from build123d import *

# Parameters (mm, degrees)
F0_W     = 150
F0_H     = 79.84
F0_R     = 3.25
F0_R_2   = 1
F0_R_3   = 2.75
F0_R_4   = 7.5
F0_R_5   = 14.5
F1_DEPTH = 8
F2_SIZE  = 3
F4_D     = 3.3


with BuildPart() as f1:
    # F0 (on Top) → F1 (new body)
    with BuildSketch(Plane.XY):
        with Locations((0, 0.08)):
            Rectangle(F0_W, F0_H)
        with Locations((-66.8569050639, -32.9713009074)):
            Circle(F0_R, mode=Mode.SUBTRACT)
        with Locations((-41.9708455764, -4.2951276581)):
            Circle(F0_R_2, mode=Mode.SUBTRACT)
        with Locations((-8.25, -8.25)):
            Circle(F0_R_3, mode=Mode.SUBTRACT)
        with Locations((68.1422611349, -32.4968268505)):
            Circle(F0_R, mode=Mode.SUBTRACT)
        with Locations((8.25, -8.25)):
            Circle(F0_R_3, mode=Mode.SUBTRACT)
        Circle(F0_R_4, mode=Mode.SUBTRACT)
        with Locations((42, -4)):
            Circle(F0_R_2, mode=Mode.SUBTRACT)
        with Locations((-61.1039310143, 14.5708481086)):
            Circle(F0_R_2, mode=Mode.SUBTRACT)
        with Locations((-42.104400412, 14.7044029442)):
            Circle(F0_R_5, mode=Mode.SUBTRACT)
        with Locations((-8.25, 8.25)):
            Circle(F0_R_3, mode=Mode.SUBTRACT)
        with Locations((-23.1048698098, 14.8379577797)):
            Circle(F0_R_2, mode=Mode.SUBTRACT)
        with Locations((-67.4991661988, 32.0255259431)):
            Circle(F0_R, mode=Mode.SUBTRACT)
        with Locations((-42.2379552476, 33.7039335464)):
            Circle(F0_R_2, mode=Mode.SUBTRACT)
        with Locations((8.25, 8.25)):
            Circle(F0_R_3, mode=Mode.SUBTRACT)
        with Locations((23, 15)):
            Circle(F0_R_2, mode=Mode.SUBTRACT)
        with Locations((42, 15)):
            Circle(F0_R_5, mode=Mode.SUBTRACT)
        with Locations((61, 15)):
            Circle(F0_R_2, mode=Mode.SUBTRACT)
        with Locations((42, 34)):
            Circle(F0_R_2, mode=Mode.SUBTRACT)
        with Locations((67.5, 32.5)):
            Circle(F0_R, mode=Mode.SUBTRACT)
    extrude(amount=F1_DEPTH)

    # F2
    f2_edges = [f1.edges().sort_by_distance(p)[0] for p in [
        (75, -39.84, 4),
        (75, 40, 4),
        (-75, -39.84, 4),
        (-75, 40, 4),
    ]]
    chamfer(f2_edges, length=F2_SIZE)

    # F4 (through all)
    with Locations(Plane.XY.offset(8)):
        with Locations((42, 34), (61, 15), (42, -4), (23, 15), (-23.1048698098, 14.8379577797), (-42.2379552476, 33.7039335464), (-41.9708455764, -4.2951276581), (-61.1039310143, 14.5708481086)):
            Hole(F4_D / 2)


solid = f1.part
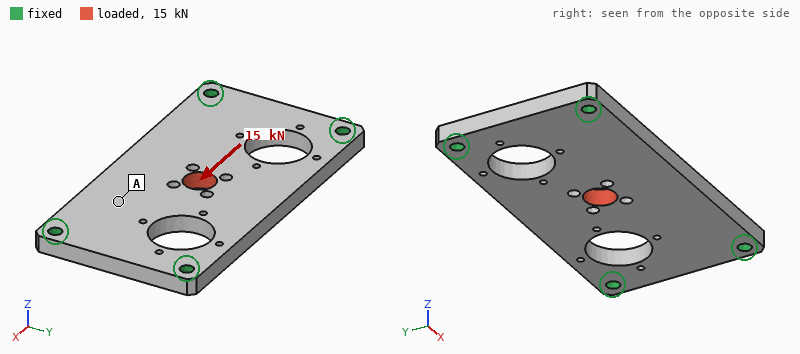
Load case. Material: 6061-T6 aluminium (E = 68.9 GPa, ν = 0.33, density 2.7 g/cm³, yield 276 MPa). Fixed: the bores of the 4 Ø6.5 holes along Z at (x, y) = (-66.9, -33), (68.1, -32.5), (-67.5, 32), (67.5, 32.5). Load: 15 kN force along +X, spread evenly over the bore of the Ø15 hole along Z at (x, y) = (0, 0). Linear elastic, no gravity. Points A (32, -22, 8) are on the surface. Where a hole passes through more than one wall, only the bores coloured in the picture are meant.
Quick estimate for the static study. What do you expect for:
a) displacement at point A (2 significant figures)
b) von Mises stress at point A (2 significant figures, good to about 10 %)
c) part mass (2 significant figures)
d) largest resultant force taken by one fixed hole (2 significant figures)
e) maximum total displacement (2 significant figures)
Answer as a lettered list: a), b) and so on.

a) 13 µm
b) 17 MPa
c) 220 g
d) 5.2 kN
e) 39 µm
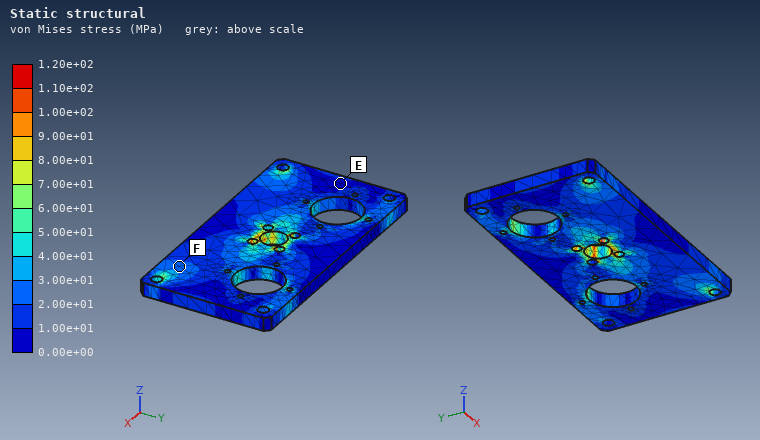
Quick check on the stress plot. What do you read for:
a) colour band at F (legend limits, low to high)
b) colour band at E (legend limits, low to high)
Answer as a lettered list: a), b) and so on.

a) 2.00e+01 to 3.00e+01 MPa
b) 0.00e+00 to 1.00e+01 MPa
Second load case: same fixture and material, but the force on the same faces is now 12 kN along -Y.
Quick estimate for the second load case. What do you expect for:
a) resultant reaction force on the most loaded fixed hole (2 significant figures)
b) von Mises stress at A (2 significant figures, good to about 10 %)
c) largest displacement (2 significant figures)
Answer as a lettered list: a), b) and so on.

a) 5.3 kN
b) 27 MPa
c) 68 µm
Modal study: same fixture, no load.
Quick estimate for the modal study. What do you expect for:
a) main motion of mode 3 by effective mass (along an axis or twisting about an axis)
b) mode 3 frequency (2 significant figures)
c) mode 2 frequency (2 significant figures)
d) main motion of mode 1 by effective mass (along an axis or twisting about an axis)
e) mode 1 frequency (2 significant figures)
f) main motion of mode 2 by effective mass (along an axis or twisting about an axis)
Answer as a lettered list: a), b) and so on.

a) twisting about Y
b) 5300 Hz
c) 3000 Hz
d) along Z
e) 1900 Hz
f) twisting about X
